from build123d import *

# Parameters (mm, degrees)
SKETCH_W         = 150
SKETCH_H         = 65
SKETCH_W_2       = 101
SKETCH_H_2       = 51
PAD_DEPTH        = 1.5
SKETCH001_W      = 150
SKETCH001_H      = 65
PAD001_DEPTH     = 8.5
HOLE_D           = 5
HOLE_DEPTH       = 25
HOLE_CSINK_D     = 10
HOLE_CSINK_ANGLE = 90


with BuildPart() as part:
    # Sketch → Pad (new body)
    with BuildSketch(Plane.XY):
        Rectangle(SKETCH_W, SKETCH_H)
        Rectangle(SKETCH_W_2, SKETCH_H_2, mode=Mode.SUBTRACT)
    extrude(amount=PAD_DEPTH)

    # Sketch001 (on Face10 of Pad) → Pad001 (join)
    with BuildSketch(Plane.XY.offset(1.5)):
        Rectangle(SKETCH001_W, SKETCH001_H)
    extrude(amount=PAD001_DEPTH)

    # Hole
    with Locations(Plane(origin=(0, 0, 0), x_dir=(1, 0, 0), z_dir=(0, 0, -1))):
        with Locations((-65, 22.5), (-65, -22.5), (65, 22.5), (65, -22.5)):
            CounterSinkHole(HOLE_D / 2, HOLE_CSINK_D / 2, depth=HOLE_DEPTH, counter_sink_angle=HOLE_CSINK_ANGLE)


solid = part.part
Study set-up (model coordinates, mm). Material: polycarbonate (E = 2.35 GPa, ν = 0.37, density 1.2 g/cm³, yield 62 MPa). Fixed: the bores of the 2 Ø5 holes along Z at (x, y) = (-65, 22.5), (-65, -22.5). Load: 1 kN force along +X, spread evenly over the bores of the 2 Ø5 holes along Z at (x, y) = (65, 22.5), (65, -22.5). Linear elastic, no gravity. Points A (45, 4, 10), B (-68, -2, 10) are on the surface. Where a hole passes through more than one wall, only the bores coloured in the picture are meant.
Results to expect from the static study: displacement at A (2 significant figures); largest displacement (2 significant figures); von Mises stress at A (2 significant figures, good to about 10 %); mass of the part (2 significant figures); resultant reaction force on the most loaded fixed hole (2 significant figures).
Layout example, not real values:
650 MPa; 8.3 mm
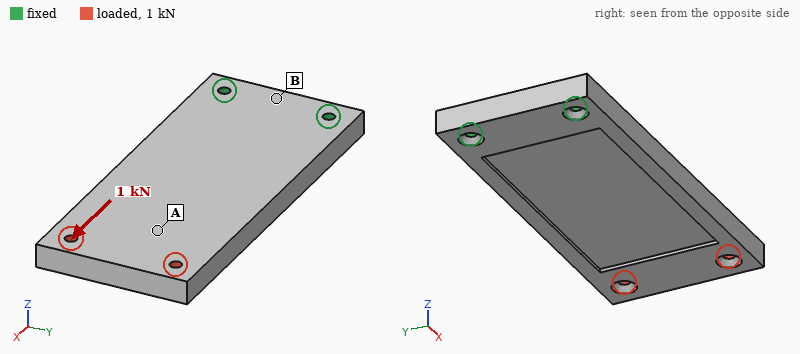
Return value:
0.51 mm; 0.81 mm; 2.0 MPa; 110 g; 510 N
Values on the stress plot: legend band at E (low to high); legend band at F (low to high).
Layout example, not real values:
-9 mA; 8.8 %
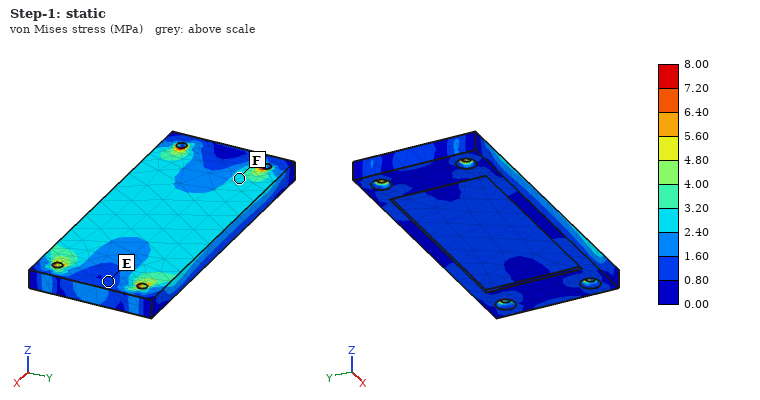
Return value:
0.80 to 1.60 MPa; 2.40 to 3.20 MPa
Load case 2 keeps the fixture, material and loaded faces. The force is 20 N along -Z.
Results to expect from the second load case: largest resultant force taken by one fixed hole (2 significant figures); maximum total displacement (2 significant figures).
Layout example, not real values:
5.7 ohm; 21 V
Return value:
15 N; 1.9 mm
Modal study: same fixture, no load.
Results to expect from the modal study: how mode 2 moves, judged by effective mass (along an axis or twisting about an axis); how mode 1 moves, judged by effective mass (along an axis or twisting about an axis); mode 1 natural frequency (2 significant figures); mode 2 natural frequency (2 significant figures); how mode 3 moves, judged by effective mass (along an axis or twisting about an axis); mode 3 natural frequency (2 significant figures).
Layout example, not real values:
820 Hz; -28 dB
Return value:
twisting about X; along Z; 98 Hz; 420 Hz; along Z; 610 Hz
